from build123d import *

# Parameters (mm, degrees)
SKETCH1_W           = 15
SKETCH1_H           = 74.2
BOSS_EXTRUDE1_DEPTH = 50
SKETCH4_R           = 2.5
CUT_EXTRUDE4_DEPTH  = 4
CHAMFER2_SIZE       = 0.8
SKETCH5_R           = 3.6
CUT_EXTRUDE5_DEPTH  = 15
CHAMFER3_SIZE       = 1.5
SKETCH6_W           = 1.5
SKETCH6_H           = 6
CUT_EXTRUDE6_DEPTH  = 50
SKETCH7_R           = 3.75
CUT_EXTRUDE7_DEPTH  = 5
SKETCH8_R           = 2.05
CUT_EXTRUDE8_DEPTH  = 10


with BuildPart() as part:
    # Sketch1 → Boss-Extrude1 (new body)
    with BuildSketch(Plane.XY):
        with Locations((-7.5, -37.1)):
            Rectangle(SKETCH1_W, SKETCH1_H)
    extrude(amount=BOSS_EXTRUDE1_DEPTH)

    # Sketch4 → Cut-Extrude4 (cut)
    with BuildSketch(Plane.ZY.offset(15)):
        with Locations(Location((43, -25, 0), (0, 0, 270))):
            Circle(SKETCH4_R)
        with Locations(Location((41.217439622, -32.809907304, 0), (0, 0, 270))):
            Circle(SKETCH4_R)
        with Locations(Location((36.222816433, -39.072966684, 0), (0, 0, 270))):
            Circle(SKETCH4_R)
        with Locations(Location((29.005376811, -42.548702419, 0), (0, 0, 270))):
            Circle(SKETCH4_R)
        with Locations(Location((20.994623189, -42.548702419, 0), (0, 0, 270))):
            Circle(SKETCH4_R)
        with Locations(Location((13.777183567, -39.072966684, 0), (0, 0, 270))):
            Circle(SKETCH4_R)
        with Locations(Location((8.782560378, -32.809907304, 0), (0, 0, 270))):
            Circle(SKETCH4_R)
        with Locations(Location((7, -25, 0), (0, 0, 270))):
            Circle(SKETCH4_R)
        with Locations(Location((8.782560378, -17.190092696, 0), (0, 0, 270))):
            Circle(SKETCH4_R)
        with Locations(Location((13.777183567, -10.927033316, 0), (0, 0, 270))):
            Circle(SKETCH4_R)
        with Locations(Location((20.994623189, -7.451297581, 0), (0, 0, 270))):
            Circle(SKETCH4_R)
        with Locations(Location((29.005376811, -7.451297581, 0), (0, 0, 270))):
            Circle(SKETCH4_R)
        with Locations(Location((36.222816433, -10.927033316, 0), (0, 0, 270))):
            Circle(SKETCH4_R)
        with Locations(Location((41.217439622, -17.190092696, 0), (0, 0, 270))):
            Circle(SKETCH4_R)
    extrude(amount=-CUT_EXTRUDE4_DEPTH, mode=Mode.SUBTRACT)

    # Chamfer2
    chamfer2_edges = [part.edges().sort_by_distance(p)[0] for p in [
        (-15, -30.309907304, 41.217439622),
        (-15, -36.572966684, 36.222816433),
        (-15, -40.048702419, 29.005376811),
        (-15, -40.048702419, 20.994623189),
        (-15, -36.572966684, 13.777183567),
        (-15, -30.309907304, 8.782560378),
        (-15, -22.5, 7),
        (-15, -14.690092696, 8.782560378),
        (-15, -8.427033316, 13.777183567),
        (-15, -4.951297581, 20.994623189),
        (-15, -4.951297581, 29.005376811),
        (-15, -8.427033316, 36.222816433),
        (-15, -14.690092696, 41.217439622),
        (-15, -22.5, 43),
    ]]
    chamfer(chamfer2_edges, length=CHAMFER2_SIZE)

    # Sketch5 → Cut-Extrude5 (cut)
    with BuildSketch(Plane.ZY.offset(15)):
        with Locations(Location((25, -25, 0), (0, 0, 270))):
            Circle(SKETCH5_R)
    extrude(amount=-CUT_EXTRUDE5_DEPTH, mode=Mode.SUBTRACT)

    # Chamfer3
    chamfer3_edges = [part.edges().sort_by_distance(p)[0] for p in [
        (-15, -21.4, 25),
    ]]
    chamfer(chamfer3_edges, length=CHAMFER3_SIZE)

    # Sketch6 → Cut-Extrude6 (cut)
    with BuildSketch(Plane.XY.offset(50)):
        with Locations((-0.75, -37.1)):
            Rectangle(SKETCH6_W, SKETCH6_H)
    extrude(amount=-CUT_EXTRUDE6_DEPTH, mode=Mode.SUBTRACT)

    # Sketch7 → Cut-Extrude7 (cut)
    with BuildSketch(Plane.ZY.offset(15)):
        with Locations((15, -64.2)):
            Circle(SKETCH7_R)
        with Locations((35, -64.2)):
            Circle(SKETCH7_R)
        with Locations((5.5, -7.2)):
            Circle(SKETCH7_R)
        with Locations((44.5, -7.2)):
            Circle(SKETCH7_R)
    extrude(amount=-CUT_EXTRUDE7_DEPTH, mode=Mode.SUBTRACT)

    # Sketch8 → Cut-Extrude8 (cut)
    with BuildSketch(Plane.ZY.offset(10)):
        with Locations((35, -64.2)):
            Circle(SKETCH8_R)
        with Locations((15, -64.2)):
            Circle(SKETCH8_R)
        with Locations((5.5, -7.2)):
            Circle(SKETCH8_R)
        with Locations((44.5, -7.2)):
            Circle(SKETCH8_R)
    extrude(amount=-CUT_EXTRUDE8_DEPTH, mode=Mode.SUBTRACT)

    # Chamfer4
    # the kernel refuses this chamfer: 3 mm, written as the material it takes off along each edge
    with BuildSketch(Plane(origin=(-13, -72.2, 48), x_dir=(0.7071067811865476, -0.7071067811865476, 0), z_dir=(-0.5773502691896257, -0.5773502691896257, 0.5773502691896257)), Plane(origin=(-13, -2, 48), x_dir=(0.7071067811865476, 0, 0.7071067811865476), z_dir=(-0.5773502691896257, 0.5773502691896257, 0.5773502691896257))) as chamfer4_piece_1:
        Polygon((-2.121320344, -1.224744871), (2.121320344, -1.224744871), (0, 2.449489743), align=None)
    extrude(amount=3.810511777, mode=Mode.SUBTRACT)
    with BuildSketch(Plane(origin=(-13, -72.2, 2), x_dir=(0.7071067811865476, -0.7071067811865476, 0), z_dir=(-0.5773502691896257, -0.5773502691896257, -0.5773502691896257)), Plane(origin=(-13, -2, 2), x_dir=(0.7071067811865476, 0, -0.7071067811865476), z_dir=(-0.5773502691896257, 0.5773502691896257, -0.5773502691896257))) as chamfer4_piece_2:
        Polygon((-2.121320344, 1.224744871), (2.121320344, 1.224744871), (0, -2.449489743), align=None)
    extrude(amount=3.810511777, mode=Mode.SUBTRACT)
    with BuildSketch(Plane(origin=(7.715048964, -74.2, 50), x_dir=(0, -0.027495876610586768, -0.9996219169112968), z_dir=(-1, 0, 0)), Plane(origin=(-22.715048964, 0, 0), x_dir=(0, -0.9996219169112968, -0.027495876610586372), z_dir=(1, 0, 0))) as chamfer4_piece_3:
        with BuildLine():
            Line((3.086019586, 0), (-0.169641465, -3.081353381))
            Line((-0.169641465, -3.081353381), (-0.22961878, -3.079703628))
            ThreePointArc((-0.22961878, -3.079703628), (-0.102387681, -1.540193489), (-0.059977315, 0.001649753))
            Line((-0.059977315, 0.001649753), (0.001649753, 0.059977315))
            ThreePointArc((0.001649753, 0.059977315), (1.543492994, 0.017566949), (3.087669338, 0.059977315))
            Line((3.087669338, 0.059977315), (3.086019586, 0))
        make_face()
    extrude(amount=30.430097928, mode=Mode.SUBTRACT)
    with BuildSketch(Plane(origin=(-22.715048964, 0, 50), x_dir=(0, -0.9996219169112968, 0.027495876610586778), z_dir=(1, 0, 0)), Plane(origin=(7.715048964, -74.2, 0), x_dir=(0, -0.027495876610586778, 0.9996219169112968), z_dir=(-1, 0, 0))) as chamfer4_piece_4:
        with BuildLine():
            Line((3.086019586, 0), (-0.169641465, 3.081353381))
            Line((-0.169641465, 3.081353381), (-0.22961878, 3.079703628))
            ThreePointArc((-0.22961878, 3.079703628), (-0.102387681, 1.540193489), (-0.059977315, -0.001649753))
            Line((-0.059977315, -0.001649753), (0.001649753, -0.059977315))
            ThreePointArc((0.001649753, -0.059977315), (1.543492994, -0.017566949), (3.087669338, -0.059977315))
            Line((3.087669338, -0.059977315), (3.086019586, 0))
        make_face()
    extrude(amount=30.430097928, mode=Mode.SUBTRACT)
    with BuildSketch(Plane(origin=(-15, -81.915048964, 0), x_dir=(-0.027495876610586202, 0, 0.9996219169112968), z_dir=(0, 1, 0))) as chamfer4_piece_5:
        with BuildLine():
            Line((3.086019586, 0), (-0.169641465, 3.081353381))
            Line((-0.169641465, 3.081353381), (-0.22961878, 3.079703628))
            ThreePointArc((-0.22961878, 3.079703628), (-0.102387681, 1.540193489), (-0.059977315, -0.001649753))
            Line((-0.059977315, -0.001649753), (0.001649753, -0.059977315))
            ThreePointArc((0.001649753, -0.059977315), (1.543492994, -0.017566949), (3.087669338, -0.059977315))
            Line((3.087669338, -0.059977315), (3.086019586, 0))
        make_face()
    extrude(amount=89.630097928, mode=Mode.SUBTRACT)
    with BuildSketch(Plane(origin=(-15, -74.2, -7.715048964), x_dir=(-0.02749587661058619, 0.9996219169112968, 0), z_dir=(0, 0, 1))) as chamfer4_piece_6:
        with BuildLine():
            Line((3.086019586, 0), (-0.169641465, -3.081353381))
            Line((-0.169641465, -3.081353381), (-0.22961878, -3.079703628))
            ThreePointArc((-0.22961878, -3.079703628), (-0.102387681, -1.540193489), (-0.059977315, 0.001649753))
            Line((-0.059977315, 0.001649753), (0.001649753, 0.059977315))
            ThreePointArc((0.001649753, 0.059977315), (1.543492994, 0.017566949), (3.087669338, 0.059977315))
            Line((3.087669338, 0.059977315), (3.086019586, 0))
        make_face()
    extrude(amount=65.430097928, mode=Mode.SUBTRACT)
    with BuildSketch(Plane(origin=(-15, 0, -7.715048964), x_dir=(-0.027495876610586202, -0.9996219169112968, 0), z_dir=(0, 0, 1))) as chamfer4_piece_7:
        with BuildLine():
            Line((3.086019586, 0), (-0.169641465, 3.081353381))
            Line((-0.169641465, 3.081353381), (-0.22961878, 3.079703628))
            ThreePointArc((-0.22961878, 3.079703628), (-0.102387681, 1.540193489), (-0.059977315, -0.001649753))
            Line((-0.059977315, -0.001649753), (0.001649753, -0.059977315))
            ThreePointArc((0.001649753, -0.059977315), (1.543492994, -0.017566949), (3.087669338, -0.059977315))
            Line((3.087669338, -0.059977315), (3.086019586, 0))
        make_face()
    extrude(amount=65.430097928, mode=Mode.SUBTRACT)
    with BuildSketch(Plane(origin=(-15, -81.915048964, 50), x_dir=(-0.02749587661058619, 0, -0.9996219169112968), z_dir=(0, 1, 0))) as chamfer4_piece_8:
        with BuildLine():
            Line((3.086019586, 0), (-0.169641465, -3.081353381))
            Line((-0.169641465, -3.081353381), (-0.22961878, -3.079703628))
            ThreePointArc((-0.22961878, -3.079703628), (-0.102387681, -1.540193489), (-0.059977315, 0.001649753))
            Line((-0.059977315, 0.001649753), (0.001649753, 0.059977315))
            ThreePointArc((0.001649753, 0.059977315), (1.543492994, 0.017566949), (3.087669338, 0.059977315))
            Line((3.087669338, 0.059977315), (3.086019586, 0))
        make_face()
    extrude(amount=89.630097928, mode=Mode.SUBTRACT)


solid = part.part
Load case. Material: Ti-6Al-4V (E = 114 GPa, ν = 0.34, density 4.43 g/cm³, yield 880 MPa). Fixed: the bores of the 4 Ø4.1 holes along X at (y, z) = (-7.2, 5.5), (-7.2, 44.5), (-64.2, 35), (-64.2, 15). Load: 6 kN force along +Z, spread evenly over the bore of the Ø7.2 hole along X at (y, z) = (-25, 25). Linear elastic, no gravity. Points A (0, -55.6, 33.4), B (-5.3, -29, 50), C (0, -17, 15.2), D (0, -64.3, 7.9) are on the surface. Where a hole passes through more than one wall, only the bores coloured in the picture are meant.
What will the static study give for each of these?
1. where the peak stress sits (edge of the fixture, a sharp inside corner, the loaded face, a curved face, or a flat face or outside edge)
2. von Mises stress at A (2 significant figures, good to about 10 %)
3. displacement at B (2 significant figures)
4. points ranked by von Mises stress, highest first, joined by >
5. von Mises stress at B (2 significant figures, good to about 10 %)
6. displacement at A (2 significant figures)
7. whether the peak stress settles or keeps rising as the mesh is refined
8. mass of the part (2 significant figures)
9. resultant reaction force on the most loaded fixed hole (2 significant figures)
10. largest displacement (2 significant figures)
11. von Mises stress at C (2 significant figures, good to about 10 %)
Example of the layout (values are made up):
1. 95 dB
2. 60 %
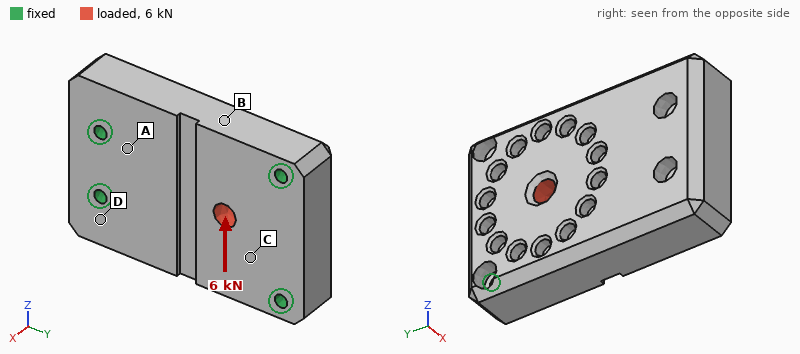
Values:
1. edge of the fixture
2. 6.8 MPa
3. 3.2 µm
4. C > B > A > D
5. 11 MPa
6. 0.98 µm
7. keeps rising
8. 220 g
9. 2.4 kN
10. 4.8 µm
11. 16 MPa
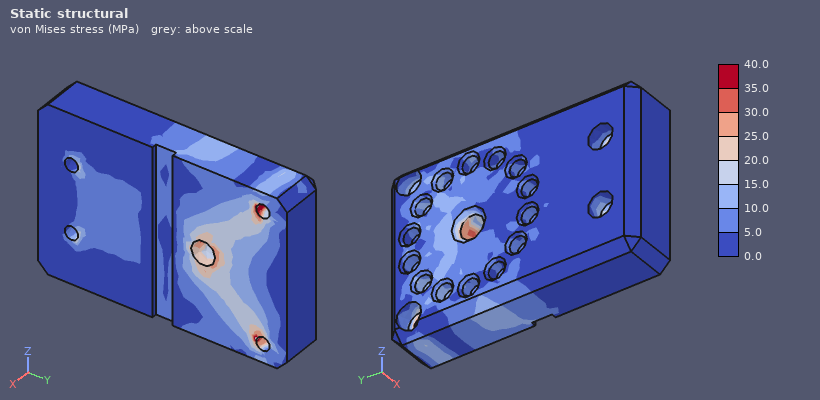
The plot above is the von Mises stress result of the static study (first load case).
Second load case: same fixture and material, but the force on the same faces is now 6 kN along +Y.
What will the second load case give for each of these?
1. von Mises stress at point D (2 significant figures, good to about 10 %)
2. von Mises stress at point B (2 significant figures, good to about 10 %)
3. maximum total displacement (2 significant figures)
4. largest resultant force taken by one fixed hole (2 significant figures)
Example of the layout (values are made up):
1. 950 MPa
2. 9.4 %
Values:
1. 2.8 MPa
2. 2.8 MPa
3. 3.5 µm
4. 1.8 kN
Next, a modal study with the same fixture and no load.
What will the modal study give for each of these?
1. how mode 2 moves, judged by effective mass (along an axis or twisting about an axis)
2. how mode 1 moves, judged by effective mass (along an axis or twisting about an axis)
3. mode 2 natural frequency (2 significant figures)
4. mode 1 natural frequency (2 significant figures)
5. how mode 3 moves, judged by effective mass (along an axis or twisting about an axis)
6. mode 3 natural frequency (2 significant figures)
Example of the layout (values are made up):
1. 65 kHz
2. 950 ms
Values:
1. twisting about Y
2. along X
3. 15 kHz
4. 12 kHz
5. along Z
6. 20 kHz
